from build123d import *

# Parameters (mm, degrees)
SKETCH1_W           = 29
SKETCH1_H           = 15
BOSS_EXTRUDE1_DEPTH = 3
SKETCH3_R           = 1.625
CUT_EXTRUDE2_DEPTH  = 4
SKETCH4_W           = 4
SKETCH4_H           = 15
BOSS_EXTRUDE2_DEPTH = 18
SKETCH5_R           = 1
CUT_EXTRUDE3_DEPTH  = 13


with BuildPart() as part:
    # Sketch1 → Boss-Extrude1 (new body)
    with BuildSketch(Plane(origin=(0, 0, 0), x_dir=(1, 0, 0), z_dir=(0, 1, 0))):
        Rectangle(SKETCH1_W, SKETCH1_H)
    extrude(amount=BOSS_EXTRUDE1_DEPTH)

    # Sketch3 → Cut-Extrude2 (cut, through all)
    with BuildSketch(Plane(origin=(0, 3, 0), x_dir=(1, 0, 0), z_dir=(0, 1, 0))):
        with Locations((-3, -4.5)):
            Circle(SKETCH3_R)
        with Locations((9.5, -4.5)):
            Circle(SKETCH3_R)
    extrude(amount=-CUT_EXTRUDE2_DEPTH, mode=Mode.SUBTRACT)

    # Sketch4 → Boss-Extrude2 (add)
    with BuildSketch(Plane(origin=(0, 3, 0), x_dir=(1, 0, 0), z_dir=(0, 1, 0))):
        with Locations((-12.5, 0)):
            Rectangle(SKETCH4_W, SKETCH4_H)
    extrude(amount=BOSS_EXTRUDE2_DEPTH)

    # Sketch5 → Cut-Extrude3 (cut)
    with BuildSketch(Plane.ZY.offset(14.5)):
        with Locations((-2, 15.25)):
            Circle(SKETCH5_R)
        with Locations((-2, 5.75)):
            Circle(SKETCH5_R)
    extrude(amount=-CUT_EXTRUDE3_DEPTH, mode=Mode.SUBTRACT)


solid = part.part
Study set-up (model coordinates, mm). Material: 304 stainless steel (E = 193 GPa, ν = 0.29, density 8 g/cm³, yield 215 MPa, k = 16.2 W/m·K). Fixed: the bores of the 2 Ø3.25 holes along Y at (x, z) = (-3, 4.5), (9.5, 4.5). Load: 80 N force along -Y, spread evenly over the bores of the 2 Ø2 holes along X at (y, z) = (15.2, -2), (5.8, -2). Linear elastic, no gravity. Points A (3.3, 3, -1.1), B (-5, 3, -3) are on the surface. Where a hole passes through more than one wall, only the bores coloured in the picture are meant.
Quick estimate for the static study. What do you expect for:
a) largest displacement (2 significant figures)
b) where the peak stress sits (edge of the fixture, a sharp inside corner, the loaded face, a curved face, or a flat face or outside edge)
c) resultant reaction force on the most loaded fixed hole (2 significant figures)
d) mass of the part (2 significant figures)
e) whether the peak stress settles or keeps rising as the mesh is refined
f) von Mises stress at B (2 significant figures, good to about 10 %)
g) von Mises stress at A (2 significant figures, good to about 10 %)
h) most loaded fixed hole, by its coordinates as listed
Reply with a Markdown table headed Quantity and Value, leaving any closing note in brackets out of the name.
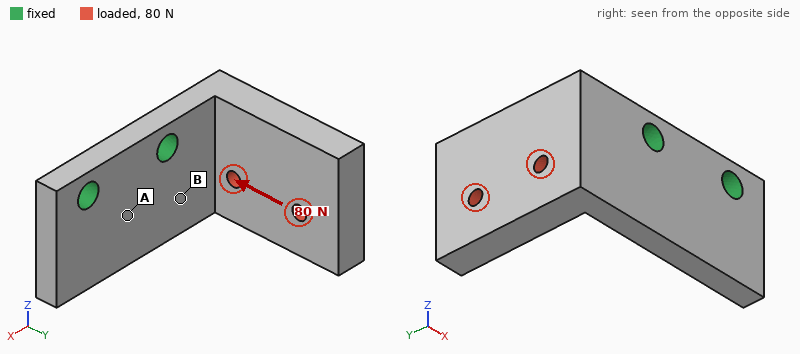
| Quantity | Value |
|---|---|
| largest displacement | 17 µm |
| where the peak stress sits | edge of the fixture |
| resultant reaction force on the most loaded fixed hole | 99 N |
| mass of the part | 18 g |
| whether the peak stress settles or keeps rising as the mesh is refined | keeps rising |
| von Mises stress at B | 18 MPa |
| von Mises stress at A | 7.9 MPa |
| most loaded fixed hole, by its coordinates as listed | (-3, 4.5) |
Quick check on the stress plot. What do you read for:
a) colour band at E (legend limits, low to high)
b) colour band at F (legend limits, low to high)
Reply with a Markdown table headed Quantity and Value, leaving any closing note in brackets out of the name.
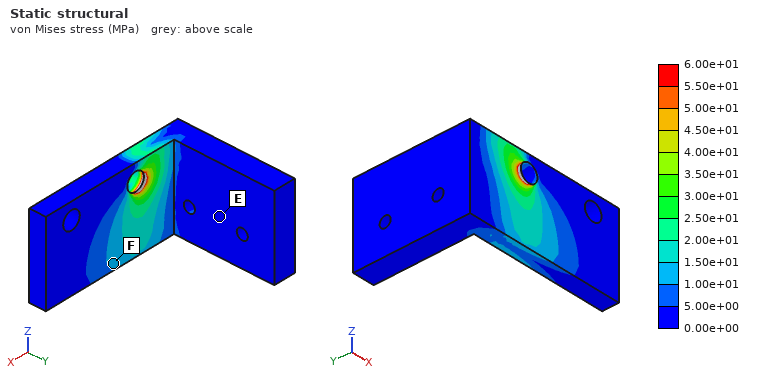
| Quantity | Value |
|---|---|
| colour band at E | 0.00e+00 to 5.00e+00 MPa |
| colour band at F | 1.00e+01 to 1.50e+01 MPa |
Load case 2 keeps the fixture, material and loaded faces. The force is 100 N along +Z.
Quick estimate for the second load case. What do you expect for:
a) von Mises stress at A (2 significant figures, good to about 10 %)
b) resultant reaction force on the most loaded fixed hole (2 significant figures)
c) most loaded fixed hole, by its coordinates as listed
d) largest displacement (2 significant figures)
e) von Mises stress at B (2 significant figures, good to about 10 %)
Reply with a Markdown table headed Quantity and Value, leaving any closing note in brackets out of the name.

| Quantity | Value |
|---|---|
| von Mises stress at A | 8.8 MPa |
| resultant reaction force on the most loaded fixed hole | 150 N |
| most loaded fixed hole, by its coordinates as listed | (-3, 4.5) |
| largest displacement | 19 µm |
| von Mises stress at B | 19 MPa |
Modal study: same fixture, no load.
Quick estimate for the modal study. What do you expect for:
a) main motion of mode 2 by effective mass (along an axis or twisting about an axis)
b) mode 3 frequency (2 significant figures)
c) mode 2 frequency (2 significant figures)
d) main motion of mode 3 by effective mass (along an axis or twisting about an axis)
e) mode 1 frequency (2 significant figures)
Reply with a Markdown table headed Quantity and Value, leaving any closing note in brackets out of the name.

| Quantity | Value |
|---|---|
| main motion of mode 2 by effective mass | along Z |
| mode 3 frequency | 12 kHz |
| mode 2 frequency | 4500 Hz |
| main motion of mode 3 by effective mass | along Y |
| mode 1 frequency | 3200 Hz |
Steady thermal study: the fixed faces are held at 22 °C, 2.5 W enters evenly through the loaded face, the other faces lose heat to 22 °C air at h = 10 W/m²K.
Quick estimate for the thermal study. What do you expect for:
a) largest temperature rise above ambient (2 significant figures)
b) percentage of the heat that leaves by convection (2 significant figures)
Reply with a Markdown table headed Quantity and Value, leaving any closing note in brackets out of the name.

| Quantity | Value |
|---|---|
| largest temperature rise above ambient | 53 K |
| percentage of the heat that leaves by convection | 17 % |
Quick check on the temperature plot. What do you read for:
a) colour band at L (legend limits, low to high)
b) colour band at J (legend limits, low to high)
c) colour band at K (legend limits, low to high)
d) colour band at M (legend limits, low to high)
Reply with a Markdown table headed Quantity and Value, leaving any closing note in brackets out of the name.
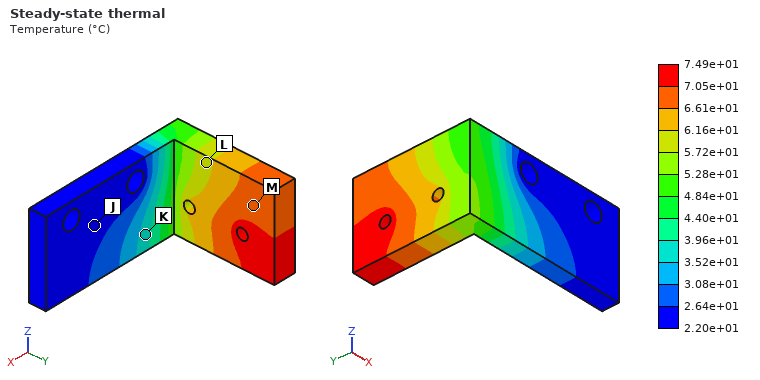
| Quantity | Value |
|---|---|
| colour band at L | 5.72e+01 to 6.16e+01 °C |
| colour band at J | 2.20e+01 to 2.64e+01 °C |
| colour band at K | 3.52e+01 to 3.96e+01 °C |
| colour band at M | 6.61e+01 to 7.05e+01 °C |
